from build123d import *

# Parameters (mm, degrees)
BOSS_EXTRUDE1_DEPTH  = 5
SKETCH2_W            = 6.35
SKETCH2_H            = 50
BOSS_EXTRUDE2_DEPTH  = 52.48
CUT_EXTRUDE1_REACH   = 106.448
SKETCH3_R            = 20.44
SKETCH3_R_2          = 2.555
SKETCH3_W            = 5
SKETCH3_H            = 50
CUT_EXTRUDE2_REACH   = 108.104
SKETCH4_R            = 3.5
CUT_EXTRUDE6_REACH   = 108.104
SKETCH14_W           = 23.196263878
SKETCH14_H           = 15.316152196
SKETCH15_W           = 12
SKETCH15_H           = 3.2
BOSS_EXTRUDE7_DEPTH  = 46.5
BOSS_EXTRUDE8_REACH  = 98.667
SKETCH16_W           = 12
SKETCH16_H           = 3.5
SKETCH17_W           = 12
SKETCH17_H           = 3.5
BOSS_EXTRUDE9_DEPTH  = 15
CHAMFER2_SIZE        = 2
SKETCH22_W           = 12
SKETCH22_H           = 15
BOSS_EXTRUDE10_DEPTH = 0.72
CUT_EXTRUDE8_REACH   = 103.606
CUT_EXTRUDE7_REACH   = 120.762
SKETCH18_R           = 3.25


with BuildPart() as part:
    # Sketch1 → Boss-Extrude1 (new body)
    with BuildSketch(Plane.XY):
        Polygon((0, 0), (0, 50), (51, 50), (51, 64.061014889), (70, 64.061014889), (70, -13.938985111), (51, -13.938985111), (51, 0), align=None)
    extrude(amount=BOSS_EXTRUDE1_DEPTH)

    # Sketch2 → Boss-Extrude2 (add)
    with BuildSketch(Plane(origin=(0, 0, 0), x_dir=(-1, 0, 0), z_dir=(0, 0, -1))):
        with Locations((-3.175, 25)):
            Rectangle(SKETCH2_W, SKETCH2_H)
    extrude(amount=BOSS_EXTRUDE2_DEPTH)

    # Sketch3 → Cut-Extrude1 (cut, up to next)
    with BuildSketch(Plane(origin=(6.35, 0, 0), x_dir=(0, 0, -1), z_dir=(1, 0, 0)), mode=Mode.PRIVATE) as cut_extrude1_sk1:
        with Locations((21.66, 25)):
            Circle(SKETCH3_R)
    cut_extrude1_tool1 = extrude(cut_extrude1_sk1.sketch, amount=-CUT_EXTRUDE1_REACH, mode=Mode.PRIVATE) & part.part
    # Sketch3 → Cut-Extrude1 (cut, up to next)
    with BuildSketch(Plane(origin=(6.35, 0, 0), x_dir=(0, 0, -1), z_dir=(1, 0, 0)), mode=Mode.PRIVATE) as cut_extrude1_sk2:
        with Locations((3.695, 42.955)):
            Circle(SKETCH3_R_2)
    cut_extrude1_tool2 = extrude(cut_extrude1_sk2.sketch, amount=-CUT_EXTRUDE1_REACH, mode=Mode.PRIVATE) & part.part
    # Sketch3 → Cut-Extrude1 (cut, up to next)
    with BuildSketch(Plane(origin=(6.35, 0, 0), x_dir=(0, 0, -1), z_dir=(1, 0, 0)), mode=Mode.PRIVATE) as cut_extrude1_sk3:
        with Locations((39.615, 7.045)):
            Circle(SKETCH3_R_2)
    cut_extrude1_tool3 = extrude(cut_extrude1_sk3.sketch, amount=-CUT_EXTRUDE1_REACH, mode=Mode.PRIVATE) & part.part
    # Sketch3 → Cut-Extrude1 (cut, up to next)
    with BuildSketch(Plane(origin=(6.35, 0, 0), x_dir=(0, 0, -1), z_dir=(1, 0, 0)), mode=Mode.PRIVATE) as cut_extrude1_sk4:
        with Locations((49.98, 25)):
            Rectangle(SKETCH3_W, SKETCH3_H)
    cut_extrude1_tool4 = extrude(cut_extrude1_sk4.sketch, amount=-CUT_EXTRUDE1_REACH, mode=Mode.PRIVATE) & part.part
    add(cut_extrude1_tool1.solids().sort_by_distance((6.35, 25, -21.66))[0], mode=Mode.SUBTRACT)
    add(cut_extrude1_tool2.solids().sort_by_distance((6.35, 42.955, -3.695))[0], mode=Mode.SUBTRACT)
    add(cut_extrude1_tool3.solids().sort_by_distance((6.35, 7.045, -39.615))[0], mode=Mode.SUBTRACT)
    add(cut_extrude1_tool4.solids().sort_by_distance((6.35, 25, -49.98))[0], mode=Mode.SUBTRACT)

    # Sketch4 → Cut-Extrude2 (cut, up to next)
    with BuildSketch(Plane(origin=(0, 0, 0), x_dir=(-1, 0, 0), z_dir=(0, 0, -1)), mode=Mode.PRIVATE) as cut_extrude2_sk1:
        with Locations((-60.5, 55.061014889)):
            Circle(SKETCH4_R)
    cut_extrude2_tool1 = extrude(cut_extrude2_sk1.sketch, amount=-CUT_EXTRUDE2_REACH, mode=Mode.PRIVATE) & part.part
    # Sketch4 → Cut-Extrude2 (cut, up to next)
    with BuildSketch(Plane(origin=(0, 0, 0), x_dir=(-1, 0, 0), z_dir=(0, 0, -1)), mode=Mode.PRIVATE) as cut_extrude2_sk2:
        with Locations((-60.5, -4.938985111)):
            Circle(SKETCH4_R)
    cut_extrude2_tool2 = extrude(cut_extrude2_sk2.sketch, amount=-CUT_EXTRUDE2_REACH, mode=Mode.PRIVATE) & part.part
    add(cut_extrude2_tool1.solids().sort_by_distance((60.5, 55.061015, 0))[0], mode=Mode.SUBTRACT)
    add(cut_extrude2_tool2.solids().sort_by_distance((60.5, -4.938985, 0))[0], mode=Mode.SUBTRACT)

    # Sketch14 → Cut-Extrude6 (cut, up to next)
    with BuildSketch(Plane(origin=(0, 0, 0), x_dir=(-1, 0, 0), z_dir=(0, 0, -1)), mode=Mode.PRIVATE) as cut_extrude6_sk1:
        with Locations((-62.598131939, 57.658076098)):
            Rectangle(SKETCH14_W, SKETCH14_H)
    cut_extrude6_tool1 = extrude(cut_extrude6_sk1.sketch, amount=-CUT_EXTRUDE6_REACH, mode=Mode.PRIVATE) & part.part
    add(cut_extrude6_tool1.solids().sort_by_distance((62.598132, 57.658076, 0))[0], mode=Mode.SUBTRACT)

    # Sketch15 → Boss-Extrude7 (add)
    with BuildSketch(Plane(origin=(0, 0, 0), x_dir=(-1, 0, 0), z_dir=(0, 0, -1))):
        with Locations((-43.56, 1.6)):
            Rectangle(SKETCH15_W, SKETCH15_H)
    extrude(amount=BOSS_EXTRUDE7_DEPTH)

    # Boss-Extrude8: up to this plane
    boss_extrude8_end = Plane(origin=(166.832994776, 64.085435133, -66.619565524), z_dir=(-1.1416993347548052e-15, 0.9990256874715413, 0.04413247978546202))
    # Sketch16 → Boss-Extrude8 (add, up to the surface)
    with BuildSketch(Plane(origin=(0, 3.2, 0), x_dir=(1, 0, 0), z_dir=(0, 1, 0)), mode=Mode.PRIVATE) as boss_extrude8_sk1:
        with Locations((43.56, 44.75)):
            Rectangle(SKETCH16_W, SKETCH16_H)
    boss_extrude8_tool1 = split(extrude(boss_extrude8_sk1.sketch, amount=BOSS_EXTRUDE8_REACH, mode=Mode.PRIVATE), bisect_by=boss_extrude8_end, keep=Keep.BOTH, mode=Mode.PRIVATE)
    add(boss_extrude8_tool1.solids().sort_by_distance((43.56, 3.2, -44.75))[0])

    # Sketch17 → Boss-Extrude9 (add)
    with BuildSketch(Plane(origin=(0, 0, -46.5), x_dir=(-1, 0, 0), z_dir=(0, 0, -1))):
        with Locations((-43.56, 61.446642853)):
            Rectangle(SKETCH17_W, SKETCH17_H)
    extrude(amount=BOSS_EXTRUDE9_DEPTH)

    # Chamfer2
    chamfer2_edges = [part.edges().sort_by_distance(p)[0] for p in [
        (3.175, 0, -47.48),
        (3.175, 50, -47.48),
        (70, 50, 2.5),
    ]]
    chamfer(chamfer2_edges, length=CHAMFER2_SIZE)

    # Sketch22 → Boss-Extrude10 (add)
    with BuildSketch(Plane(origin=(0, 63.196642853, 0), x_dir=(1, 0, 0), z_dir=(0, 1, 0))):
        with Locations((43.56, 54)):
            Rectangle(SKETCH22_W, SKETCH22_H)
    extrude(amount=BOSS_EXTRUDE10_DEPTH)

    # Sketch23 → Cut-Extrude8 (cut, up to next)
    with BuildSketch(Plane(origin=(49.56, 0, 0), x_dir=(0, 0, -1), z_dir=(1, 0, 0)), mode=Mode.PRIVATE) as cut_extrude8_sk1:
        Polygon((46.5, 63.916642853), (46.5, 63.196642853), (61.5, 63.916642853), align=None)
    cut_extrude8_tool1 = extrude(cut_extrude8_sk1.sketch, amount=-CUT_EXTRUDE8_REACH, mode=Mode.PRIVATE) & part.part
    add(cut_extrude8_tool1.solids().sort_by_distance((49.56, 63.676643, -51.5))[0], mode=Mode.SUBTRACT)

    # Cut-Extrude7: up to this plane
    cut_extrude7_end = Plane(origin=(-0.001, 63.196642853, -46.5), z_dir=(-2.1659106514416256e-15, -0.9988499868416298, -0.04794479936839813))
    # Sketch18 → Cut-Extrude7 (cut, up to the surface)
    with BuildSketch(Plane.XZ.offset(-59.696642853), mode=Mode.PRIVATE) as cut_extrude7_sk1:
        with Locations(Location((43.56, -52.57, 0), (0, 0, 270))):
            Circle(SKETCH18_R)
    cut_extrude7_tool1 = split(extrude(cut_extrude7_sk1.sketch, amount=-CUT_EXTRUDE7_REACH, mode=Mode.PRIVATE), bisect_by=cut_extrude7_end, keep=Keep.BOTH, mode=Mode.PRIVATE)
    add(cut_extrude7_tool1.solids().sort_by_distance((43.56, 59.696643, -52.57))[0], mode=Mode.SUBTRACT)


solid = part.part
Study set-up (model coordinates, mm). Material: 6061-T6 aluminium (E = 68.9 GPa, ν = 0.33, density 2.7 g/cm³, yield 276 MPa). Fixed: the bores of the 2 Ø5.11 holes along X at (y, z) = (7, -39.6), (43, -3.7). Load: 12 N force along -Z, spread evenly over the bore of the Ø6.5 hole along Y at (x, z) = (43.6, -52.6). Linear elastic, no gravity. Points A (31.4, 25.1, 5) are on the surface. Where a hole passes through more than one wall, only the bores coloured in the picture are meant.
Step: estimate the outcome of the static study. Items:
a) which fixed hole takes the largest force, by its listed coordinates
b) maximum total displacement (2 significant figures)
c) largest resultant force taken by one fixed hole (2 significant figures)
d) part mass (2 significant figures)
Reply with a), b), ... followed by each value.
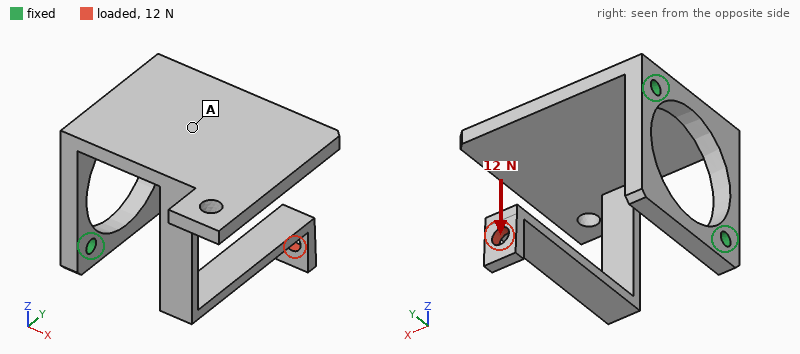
a) (43, -3.7)
b) 1.4 mm
c) 19 N
d) 81 g
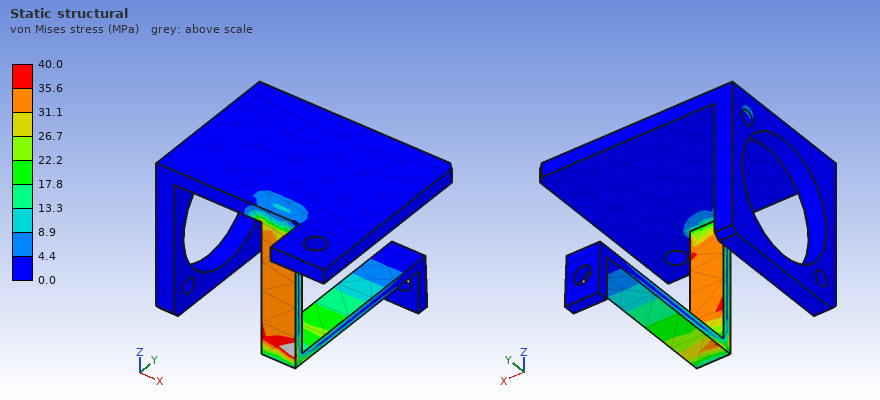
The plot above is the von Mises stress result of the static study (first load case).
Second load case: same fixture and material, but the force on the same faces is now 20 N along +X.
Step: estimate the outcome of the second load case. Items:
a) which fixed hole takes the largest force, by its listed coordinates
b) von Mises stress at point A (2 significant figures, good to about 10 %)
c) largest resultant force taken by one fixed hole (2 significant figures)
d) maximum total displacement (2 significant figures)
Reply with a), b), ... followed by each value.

a) (43, -3.7)
b) 4.9 MPa
c) 12 N
d) 1.3 mm
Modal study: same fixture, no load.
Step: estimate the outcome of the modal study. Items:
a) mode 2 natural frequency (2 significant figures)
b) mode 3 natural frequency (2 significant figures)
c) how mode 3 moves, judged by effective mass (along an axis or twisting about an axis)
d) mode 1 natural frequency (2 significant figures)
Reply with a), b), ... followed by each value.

a) 310 Hz
b) 570 Hz
c) along Z
d) 220 Hz
